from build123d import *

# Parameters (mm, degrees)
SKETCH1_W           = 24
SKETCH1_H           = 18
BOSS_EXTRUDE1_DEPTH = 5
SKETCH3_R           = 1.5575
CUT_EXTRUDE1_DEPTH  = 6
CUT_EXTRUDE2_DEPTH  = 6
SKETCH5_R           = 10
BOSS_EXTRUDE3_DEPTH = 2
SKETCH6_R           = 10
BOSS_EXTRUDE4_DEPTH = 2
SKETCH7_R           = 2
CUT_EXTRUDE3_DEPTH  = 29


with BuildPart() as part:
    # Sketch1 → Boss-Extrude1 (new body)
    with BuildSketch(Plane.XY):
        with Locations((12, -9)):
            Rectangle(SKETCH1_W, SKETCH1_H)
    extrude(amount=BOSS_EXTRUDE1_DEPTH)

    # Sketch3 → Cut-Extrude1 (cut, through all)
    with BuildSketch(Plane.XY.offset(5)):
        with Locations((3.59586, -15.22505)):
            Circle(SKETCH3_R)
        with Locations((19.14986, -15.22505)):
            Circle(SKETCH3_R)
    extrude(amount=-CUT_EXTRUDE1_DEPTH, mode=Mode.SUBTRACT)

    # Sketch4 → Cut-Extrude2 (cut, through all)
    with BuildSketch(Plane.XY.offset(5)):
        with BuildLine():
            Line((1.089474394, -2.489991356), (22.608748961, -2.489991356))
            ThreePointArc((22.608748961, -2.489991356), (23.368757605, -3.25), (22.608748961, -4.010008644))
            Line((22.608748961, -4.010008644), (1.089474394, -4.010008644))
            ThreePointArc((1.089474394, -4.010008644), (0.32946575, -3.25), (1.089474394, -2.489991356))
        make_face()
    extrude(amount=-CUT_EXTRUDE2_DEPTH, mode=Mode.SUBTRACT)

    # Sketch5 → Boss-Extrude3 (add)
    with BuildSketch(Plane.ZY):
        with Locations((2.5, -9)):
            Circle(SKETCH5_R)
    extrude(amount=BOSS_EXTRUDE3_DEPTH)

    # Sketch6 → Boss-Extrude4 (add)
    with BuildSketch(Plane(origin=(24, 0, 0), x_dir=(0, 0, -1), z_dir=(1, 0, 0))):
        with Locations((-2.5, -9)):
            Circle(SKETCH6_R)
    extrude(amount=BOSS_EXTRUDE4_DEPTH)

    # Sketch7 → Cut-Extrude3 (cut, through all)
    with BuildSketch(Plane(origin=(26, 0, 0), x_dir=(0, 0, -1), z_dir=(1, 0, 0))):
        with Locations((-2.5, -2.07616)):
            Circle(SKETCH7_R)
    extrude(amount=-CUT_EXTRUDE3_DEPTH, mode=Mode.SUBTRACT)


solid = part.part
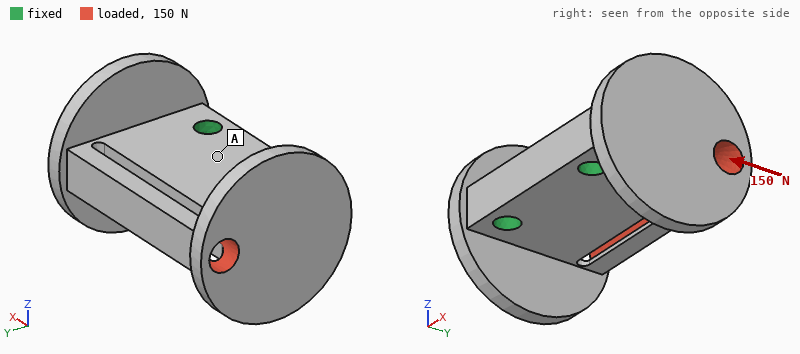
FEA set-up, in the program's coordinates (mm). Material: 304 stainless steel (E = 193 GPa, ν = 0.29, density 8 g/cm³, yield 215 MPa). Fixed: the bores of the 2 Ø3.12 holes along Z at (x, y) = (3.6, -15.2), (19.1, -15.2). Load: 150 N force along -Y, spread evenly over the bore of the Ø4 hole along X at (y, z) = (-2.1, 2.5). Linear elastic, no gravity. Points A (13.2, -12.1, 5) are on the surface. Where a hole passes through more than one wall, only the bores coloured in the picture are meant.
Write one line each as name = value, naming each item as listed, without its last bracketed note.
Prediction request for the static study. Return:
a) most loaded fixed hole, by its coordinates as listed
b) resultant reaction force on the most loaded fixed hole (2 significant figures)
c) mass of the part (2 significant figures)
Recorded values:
most loaded fixed hole, by its coordinates as listed = (19.1, -15.2)
resultant reaction force on the most loaded fixed hole = 83 N
mass of the part = 23 g
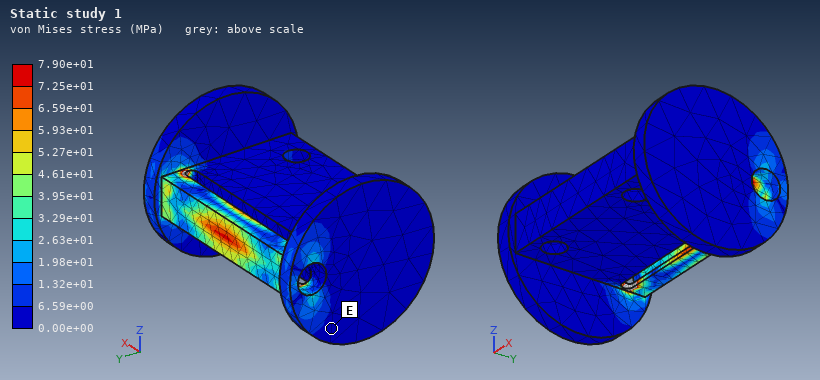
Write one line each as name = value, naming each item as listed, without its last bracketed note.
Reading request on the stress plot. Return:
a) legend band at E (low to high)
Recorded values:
legend band at E = 0.00e+00 to 6.59e+00 MPa
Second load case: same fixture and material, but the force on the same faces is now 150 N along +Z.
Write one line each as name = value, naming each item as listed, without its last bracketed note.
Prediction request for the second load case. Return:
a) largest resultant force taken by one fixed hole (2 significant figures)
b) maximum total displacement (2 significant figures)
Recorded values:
largest resultant force taken by one fixed hole = 79 N
maximum total displacement = 20 µm
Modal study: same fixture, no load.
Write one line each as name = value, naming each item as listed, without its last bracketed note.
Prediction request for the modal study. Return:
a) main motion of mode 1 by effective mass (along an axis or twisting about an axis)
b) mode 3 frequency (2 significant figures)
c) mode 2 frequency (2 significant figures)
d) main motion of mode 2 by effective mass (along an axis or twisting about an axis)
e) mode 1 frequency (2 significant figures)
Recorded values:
main motion of mode 1 by effective mass = along Z
mode 3 frequency = 17 kHz
mode 2 frequency = 15 kHz
main motion of mode 2 by effective mass = twisting about Y
mode 1 frequency = 14 kHz
